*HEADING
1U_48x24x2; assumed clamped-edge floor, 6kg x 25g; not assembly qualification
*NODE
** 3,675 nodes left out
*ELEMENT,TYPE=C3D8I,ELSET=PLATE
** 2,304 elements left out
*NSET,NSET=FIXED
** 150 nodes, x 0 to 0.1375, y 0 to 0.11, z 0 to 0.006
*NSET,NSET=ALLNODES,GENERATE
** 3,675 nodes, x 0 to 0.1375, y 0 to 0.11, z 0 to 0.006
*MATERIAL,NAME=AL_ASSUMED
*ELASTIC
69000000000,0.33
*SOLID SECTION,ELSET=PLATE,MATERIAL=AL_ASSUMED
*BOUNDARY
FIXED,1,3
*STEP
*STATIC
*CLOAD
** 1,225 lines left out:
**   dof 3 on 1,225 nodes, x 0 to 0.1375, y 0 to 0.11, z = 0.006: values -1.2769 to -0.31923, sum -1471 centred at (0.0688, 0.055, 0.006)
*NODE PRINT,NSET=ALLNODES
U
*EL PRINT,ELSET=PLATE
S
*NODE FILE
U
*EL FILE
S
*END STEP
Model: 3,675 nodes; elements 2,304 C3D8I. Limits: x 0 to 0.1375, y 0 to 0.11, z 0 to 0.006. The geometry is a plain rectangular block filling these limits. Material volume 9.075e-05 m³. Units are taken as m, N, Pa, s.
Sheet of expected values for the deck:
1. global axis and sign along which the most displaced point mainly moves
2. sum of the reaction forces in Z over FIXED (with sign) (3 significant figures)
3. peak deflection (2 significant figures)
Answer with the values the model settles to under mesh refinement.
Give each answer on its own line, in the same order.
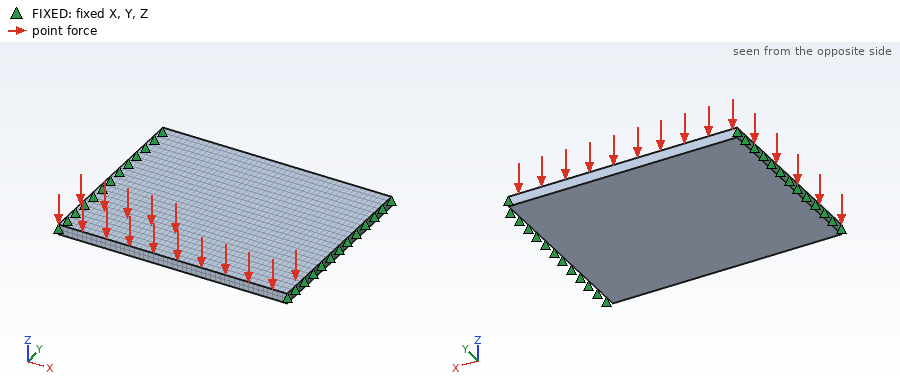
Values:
-Z
1470 N
7.5e-05 m
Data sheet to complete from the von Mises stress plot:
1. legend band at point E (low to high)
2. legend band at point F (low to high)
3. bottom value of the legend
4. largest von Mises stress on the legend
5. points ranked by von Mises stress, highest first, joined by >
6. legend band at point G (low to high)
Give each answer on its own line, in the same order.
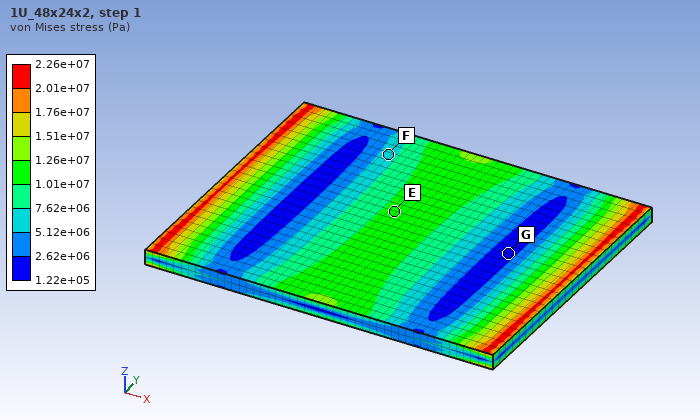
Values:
1.01e+07 to 1.26e+07 Pa
5.12e+06 to 7.62e+06 Pa
1.22e+05 Pa
2.26e+07 Pa
E > F > G
1.22e+05 to 2.62e+06 Pa
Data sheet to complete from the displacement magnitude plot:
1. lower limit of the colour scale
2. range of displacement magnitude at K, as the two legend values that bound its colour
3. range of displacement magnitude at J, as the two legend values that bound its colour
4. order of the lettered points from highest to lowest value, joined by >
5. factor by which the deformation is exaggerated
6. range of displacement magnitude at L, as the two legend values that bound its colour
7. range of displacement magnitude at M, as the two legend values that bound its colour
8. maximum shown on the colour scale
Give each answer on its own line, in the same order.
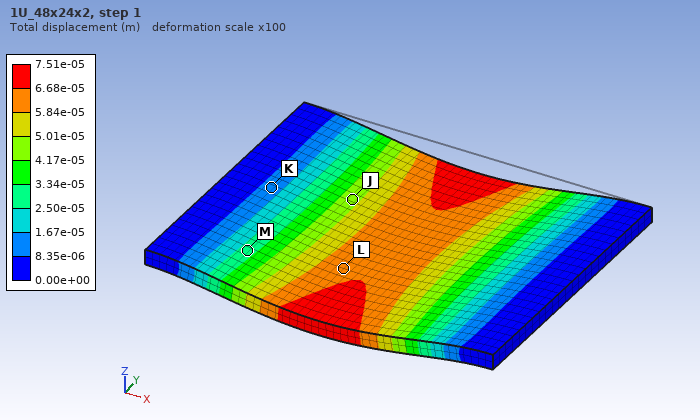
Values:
0.00e+00 m
8.35e-06 to 1.67e-05 m
4.17e-05 to 5.01e-05 m
L > J > M > K
100
5.84e-05 to 6.68e-05 m
2.50e-05 to 3.34e-05 m
7.51e-05 m
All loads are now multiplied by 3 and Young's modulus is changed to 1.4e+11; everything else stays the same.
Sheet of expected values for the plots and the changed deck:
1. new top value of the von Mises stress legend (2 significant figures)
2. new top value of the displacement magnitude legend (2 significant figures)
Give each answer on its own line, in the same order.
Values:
6.8e+07 Pa
1.1e-04 m
